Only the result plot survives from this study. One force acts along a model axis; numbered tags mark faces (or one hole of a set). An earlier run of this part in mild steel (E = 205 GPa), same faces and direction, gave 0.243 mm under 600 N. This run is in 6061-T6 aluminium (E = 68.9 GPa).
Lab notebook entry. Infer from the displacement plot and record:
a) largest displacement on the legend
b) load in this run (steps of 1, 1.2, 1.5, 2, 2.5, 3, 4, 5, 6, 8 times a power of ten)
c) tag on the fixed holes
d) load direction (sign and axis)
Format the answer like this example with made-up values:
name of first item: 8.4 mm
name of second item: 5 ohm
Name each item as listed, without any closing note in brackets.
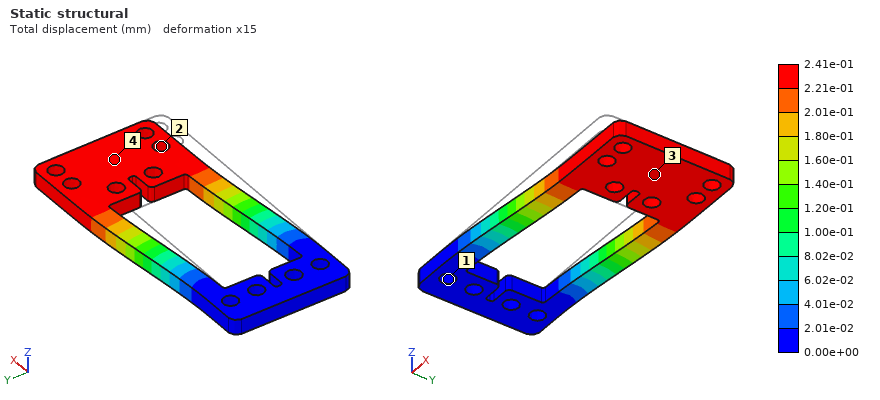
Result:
largest displacement on the legend: 2.41e-01 mm
load in this run: 200 N
tag on the fixed holes: 1
load direction: +Y
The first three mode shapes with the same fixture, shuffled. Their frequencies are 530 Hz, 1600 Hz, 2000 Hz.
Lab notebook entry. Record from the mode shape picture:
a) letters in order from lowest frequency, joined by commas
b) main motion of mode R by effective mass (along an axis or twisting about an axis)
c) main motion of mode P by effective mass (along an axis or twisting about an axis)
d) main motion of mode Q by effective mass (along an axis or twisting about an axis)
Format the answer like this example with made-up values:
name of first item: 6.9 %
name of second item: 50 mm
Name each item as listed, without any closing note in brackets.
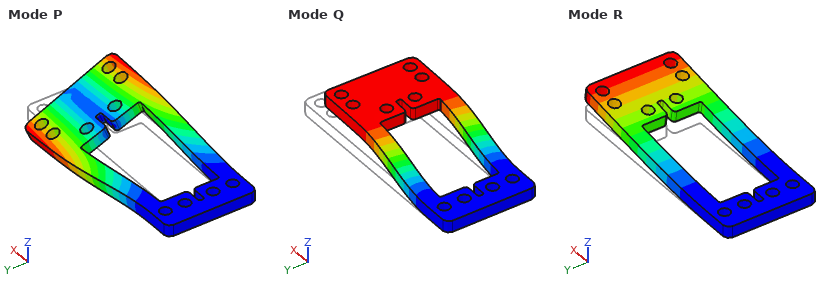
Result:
letters in order from lowest frequency, joined by commas: R, Q, P
main motion of mode R by effective mass: along Z
main motion of mode P by effective mass: twisting about X
main motion of mode Q by effective mass: along Y
